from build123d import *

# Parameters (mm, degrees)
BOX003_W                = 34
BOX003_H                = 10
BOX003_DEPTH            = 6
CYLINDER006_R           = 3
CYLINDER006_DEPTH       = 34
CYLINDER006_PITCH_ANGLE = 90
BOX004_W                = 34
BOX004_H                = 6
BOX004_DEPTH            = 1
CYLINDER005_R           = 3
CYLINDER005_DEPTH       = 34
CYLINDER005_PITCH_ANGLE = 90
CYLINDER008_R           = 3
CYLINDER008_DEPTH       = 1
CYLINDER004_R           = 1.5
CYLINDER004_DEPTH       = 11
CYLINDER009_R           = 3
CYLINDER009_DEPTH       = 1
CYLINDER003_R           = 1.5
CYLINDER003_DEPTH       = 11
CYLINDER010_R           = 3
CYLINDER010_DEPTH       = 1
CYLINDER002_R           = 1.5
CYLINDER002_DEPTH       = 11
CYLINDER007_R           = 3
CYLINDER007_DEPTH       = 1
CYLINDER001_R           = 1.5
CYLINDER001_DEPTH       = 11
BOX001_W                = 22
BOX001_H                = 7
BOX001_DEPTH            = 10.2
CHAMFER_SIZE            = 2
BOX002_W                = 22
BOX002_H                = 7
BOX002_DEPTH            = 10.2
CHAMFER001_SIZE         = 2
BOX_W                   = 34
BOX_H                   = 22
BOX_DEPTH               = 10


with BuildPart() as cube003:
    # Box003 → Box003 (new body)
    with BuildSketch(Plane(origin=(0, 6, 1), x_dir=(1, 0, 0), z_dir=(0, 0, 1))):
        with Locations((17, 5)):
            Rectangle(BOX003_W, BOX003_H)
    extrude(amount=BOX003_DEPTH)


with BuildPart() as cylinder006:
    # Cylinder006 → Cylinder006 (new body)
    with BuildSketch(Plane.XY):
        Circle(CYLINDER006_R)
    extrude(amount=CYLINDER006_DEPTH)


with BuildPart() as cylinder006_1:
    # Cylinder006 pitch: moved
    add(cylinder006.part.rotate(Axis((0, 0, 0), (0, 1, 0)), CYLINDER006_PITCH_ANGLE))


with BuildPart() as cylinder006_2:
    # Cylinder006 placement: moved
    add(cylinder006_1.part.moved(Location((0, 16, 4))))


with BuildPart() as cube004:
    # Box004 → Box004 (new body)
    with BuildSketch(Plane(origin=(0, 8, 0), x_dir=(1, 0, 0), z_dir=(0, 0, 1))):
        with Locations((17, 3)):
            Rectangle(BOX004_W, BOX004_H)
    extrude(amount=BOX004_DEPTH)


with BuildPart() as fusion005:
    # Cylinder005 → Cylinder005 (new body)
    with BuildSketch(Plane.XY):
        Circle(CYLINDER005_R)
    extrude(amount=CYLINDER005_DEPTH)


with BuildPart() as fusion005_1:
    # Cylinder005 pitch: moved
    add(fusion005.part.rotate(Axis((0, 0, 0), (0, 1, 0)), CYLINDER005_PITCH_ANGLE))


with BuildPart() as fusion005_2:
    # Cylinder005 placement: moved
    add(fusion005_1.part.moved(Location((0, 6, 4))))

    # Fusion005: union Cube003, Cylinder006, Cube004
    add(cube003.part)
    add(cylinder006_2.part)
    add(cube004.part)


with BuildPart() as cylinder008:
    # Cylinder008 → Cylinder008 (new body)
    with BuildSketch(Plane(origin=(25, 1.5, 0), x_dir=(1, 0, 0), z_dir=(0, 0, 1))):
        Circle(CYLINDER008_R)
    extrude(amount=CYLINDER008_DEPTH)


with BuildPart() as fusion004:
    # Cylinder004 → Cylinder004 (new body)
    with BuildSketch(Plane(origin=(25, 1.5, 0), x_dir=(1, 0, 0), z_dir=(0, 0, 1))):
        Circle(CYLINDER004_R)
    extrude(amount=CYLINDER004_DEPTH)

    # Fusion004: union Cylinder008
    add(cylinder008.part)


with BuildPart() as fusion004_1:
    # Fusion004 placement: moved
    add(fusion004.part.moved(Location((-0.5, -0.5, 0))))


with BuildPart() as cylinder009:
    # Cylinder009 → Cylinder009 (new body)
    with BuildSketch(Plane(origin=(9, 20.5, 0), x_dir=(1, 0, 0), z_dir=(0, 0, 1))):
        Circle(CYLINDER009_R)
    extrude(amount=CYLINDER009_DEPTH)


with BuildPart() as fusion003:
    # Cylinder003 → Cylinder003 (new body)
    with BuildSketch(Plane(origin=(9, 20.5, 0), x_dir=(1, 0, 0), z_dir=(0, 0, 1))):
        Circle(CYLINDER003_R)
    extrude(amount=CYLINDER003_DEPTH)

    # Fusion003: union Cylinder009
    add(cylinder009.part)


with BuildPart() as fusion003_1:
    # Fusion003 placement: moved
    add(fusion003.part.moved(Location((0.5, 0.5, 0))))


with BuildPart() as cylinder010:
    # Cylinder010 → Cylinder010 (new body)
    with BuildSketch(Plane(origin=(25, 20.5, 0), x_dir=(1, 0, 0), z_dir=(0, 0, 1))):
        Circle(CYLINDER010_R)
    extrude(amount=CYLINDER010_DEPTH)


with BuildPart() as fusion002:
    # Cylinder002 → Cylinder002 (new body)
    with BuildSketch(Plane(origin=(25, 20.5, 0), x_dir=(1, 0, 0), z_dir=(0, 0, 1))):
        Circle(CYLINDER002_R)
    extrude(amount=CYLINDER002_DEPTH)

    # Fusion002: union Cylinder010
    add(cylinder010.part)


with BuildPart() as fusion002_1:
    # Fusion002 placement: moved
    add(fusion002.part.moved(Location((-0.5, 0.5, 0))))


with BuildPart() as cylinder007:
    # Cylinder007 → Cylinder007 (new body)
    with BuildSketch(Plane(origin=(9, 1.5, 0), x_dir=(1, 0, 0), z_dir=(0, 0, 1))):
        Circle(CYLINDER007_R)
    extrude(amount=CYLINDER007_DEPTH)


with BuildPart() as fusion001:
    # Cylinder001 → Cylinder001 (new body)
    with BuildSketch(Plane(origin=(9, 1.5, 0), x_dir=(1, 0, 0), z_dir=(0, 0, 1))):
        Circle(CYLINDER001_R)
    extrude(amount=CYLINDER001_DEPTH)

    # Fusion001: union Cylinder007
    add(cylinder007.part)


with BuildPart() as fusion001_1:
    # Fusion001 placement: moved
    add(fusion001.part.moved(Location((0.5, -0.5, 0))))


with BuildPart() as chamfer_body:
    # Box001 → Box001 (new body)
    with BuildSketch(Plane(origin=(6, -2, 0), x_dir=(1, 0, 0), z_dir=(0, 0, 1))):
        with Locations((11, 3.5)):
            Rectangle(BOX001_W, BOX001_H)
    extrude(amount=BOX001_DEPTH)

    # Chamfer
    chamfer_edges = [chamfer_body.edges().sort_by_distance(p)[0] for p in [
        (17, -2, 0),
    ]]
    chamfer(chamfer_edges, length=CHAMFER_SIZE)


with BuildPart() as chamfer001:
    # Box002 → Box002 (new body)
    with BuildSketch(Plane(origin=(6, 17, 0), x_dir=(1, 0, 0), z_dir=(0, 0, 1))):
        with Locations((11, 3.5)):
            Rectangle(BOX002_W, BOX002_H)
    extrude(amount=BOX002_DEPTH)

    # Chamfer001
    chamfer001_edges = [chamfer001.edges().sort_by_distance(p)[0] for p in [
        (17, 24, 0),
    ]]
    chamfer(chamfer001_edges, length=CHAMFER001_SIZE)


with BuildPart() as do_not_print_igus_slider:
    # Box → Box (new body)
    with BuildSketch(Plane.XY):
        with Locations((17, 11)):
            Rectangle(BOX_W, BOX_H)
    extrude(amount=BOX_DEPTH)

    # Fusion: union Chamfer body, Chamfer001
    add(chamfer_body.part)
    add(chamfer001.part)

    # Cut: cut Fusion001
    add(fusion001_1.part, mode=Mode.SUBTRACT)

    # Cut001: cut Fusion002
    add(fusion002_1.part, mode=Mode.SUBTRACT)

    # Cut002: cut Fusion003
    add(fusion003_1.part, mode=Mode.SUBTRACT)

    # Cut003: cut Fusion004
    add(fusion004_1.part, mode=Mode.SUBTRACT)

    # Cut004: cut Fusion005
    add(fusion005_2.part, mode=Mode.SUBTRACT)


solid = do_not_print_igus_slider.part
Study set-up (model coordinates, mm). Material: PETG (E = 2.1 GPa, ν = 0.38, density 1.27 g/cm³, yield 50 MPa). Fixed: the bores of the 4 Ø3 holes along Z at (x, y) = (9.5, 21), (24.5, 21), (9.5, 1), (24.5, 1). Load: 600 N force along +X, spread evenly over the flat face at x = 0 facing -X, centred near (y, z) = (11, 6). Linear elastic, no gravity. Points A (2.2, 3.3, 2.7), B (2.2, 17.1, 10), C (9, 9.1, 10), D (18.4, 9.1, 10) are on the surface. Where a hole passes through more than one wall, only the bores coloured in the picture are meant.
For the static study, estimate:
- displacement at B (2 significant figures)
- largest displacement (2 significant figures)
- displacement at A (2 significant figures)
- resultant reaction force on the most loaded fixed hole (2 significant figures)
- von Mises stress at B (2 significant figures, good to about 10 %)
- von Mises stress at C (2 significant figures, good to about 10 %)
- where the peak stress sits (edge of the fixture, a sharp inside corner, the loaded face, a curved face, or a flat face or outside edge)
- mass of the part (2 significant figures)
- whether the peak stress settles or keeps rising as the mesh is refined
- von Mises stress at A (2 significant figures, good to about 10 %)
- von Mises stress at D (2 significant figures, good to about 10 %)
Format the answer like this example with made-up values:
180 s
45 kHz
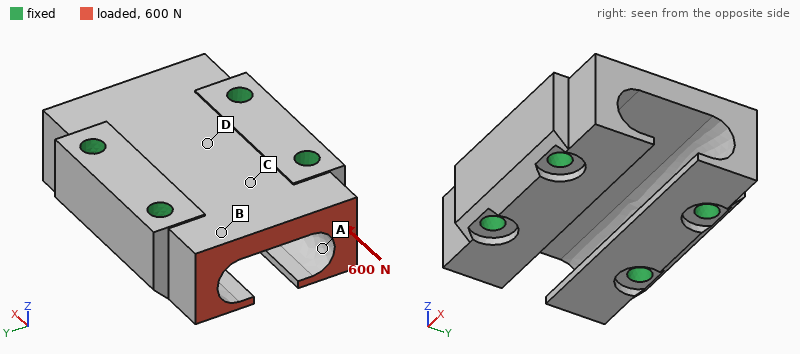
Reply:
23 µm
43 µm
23 µm
260 N
4.7 MPa
2.9 MPa
edge of the fixture
6.1 g
keeps rising
5.5 MPa
1.5 MPa
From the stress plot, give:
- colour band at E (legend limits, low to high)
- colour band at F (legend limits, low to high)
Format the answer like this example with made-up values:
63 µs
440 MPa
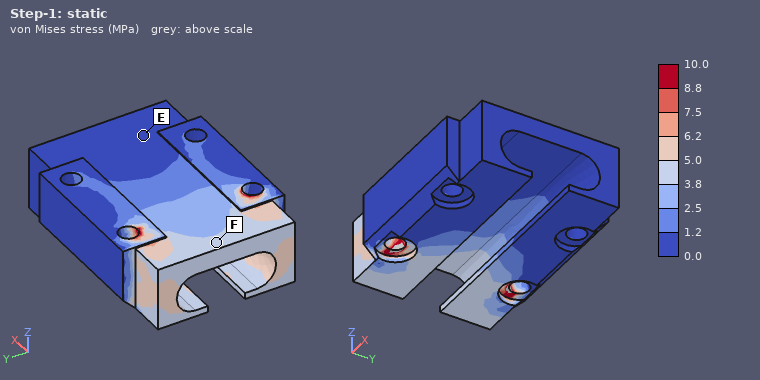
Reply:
0.0 to 1.2 MPa
3.8 to 5.0 MPa
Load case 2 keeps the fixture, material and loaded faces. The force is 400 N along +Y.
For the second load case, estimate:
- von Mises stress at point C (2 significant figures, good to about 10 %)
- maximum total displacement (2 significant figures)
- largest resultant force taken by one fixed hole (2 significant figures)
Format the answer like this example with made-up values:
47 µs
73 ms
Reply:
4.8 MPa
0.17 mm
250 N
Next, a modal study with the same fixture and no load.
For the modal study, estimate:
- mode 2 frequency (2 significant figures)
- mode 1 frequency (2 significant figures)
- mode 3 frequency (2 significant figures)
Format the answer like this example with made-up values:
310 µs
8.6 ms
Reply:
9600 Hz
9500 Hz
11 kHz
